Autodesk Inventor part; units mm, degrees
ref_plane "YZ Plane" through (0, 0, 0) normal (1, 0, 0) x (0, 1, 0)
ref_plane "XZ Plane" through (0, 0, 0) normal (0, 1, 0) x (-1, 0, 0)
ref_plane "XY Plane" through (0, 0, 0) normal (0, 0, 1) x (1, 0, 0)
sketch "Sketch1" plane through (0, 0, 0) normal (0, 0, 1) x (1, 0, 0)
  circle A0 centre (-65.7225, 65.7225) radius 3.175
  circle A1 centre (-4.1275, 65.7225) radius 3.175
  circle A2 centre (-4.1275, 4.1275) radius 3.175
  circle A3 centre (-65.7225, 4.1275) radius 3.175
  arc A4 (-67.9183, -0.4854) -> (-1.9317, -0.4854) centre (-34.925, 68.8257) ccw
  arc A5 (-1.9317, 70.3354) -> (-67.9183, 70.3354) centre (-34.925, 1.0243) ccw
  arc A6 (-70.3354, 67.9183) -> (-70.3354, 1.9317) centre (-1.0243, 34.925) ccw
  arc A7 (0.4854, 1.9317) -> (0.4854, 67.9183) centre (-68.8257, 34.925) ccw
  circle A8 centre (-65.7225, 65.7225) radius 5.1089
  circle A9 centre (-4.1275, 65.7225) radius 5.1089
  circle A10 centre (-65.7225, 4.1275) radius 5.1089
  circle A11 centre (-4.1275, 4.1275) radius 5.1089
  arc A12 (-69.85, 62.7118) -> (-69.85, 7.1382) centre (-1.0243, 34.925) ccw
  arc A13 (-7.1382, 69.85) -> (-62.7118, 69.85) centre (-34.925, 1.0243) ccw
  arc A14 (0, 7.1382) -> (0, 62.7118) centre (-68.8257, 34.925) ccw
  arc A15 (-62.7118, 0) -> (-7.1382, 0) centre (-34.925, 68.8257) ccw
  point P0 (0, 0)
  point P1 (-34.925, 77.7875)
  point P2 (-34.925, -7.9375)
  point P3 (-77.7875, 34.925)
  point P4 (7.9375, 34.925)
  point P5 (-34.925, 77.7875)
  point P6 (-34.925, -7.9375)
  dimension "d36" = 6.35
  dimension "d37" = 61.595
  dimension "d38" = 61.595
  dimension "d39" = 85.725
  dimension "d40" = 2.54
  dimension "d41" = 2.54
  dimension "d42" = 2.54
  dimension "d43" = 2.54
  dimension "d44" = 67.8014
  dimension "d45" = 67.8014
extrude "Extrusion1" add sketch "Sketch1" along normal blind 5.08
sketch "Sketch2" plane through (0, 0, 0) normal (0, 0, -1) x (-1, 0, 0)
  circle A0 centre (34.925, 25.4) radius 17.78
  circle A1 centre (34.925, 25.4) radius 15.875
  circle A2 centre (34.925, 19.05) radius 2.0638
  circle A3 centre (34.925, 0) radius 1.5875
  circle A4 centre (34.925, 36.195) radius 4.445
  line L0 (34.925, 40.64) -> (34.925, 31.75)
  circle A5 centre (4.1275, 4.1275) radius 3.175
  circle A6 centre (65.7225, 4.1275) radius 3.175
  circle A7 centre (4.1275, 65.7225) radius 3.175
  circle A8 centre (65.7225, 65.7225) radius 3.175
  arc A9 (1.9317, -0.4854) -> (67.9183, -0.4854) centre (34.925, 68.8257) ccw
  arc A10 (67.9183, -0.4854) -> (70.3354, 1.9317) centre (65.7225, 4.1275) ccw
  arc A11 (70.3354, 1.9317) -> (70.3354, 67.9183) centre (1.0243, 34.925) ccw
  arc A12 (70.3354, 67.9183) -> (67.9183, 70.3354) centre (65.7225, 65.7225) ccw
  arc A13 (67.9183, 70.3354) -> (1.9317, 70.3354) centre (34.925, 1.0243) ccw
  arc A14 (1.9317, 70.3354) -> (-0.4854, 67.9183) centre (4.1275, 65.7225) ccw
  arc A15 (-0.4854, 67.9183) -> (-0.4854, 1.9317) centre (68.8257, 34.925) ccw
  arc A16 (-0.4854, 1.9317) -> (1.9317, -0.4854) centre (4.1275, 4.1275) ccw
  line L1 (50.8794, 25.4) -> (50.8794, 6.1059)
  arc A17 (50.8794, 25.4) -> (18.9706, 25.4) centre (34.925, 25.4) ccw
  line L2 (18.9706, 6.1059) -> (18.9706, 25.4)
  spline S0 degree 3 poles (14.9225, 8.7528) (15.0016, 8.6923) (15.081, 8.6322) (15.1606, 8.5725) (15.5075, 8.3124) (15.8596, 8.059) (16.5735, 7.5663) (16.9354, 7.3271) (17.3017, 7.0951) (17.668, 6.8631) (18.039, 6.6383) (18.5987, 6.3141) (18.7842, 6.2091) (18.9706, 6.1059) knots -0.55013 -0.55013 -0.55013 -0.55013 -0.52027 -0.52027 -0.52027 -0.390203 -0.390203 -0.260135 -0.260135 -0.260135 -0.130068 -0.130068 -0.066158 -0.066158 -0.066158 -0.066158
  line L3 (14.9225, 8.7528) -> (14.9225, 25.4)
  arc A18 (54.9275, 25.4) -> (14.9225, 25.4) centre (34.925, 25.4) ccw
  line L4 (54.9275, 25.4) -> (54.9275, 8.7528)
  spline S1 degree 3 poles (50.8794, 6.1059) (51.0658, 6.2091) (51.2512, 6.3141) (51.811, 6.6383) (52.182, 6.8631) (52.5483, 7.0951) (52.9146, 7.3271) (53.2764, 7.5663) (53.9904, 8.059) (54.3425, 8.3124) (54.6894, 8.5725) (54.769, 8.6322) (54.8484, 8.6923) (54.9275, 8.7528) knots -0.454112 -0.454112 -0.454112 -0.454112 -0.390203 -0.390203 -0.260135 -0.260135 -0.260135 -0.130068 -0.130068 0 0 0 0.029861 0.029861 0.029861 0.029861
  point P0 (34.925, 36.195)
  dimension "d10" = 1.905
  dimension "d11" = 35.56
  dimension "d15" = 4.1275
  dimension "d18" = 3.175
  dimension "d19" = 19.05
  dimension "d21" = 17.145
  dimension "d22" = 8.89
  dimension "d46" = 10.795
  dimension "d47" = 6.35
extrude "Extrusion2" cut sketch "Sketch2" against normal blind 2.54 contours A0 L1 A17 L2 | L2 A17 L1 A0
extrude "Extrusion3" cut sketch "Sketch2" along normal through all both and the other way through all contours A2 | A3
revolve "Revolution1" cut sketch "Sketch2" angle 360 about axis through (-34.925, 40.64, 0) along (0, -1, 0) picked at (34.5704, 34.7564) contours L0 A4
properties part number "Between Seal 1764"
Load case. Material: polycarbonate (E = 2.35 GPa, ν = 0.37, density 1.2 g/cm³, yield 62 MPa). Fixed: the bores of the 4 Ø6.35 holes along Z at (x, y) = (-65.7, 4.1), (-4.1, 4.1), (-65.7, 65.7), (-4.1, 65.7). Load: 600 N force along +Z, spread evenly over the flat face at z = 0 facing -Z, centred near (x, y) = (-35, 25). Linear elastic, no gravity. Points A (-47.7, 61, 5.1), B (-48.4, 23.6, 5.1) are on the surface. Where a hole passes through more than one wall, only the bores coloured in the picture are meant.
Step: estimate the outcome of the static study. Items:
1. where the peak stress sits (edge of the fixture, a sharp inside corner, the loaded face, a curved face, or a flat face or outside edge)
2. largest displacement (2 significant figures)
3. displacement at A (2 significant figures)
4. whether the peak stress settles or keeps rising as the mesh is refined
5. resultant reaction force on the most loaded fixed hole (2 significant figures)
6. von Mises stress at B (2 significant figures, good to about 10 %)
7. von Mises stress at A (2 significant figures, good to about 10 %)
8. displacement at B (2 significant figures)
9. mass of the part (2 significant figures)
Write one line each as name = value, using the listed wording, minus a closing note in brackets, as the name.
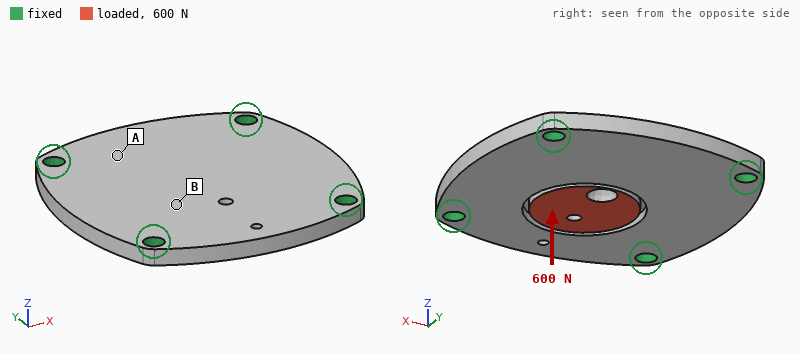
where the peak stress sits = edge of the fixture
largest displacement = 0.92 mm
displacement at A = 0.20 mm
whether the peak stress settles or keeps rising as the mesh is refined = keeps rising
resultant reaction force on the most loaded fixed hole = 230 N
von Mises stress at B = 13 MPa
von Mises stress at A = 4.9 MPa
displacement at B = 0.71 mm
mass of the part = 37 g
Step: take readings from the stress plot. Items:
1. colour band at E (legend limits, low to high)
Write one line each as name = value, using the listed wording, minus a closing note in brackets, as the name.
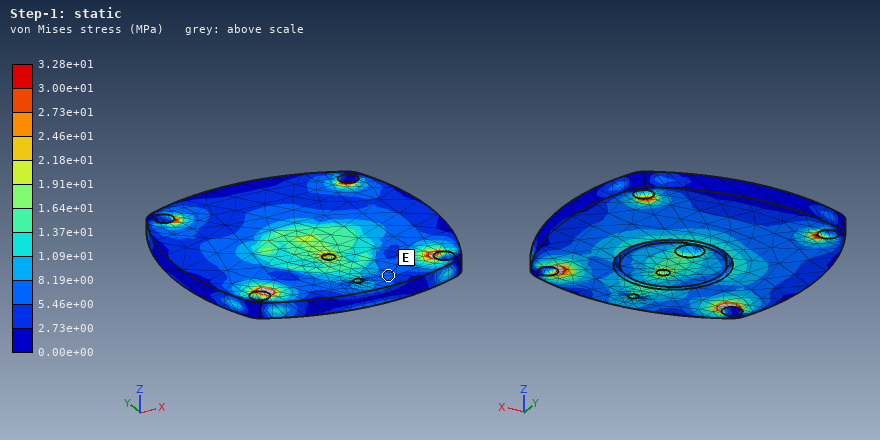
colour band at E = 5.46e+00 to 8.19e+00 MPa
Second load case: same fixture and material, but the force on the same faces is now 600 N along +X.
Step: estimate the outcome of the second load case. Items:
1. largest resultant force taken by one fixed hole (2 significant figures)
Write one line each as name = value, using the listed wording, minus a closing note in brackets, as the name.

largest resultant force taken by one fixed hole = 200 N
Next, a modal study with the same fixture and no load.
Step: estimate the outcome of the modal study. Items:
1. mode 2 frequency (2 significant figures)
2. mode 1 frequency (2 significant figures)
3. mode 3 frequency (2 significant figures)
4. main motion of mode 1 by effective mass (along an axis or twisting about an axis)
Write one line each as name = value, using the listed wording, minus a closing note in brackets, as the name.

mode 2 frequency = 2000 Hz
mode 1 frequency = 1300 Hz
mode 3 frequency = 2000 Hz
main motion of mode 1 by effective mass = along Z
